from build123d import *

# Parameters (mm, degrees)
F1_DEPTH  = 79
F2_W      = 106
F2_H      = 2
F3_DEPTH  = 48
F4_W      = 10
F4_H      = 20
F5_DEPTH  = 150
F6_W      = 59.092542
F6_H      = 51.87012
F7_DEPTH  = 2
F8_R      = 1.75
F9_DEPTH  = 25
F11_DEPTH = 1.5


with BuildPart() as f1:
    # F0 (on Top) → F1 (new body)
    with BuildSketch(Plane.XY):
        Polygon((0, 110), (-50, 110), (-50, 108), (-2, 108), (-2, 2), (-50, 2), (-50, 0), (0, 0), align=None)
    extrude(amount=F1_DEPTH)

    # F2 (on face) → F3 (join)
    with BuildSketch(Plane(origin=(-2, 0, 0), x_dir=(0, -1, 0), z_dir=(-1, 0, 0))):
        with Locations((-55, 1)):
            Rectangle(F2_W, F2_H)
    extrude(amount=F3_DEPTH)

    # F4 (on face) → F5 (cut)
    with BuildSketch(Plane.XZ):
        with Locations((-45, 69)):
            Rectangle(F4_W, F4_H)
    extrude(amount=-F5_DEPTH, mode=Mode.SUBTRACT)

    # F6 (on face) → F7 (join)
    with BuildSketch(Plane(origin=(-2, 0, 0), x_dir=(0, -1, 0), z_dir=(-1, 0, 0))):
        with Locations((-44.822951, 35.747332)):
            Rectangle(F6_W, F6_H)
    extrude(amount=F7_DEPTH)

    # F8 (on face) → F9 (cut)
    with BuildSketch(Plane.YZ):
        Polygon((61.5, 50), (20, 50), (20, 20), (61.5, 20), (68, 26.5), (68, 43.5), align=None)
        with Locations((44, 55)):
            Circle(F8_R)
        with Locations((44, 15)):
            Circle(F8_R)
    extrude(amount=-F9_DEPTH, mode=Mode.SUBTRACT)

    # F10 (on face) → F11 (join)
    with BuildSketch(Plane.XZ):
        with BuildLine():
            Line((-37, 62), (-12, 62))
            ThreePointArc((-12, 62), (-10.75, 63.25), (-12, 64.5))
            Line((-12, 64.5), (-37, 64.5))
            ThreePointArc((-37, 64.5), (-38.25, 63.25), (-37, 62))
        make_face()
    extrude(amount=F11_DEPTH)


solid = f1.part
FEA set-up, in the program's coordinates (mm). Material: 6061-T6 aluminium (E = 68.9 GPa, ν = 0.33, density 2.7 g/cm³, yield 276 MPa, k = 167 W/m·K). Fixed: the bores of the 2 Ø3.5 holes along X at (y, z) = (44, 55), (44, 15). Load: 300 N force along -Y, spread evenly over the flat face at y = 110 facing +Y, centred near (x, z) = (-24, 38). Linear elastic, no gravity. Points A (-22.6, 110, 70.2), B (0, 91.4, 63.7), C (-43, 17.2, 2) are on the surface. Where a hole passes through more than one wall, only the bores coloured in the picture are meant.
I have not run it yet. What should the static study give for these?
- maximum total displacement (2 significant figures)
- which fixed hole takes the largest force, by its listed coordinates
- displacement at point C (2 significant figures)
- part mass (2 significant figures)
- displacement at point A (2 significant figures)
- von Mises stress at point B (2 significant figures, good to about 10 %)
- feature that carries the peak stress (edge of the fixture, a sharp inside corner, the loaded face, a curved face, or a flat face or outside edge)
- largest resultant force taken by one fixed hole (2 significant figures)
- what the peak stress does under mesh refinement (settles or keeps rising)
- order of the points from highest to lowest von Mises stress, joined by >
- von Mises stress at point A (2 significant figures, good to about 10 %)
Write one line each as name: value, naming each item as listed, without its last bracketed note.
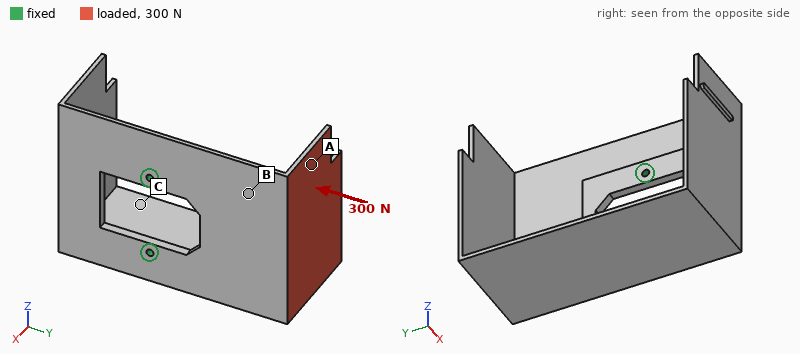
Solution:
maximum total displacement: 1.5 mm
which fixed hole takes the largest force, by its listed coordinates: (44, 55)
displacement at point C: 0.35 mm
part mass: 110 g
displacement at point A: 0.86 mm
von Mises stress at point B: 36 MPa
feature that carries the peak stress: edge of the fixture
largest resultant force taken by one fixed hole: 160 N
what the peak stress does under mesh refinement: keeps rising
order of the points from highest to lowest von Mises stress, joined by >: B > A > C
von Mises stress at point A: 19 MPa
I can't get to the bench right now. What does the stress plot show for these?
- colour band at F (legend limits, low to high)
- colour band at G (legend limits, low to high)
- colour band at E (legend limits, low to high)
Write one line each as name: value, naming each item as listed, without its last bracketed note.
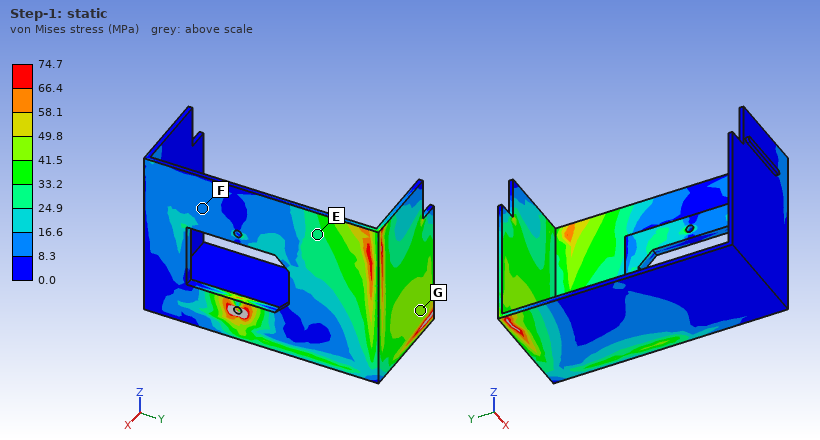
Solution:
colour band at F: 8.3 to 16.6 MPa
colour band at G: 41.5 to 49.8 MPa
colour band at E: 24.9 to 33.2 MPa
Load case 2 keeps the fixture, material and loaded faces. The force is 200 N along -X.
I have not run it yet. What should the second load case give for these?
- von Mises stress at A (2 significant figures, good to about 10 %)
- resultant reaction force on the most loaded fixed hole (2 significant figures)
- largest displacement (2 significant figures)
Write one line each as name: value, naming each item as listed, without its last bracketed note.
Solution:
von Mises stress at A: 18 MPa
resultant reaction force on the most loaded fixed hole: 110 N
largest displacement: 1.6 mm
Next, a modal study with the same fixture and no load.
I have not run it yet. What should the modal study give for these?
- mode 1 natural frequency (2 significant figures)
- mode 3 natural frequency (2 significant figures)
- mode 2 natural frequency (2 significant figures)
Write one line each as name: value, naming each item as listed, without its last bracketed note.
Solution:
mode 1 natural frequency: 360 Hz
mode 3 natural frequency: 620 Hz
mode 2 natural frequency: 450 Hz
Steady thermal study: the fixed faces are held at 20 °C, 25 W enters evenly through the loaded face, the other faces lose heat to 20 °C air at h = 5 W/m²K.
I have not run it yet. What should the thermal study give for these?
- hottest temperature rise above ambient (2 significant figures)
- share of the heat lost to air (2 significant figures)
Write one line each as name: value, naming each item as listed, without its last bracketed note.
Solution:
hottest temperature rise above ambient: 59 K
share of the heat lost to air: 15 %
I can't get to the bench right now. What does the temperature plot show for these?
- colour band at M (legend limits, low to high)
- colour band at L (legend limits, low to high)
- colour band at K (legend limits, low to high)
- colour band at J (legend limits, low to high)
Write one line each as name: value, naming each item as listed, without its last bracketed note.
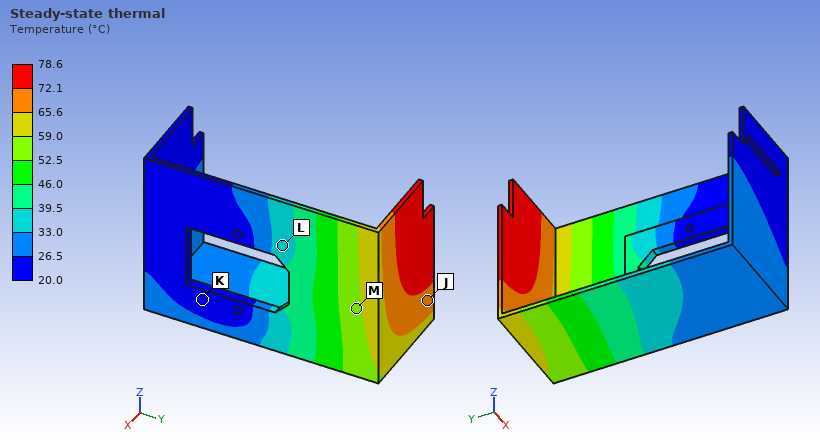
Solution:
colour band at M: 52.5 to 59.0 °C
colour band at L: 33.0 to 39.5 °C
colour band at K: 20.0 to 26.5 °C
colour band at J: 65.6 to 72.1 °C
